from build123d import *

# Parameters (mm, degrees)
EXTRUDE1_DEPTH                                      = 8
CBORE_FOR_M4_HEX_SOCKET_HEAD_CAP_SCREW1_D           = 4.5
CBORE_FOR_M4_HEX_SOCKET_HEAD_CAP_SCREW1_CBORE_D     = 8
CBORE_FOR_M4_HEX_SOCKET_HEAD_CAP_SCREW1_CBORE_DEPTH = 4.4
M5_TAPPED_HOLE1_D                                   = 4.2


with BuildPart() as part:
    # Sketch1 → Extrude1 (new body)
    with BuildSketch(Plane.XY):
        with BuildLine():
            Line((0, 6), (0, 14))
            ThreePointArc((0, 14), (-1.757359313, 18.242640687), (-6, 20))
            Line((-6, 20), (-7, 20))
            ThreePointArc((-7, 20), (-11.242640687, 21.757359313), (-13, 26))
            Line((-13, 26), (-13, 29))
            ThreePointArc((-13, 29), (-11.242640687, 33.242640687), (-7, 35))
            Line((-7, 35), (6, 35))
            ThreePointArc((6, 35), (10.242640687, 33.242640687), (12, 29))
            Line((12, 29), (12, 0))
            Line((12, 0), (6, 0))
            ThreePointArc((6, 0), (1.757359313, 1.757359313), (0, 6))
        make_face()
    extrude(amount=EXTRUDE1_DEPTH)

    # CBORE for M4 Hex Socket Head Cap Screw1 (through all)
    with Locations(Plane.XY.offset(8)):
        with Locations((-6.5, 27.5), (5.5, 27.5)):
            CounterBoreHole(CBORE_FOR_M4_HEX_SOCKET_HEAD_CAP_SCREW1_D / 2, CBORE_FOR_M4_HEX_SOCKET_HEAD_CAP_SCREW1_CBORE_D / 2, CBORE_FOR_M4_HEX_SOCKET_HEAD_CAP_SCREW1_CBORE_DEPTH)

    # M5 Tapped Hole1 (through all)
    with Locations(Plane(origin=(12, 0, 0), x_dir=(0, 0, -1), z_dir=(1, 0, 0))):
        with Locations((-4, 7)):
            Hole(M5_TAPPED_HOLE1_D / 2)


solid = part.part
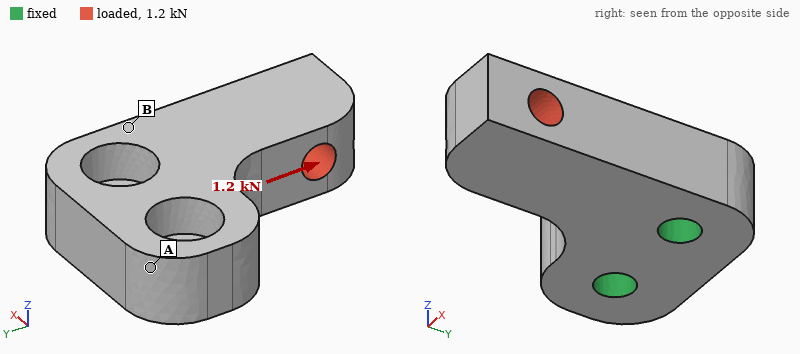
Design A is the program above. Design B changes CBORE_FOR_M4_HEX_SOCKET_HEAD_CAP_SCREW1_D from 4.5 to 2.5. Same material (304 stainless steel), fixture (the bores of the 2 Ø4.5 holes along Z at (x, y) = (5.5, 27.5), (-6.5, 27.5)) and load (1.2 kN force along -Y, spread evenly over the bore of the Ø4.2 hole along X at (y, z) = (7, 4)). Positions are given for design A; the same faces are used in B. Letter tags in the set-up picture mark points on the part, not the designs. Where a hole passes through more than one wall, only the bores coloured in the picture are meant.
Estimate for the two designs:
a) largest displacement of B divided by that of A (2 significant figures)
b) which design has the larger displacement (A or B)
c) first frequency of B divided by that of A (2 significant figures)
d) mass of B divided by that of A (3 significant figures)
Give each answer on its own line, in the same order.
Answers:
1.6
B
0.81
1.02
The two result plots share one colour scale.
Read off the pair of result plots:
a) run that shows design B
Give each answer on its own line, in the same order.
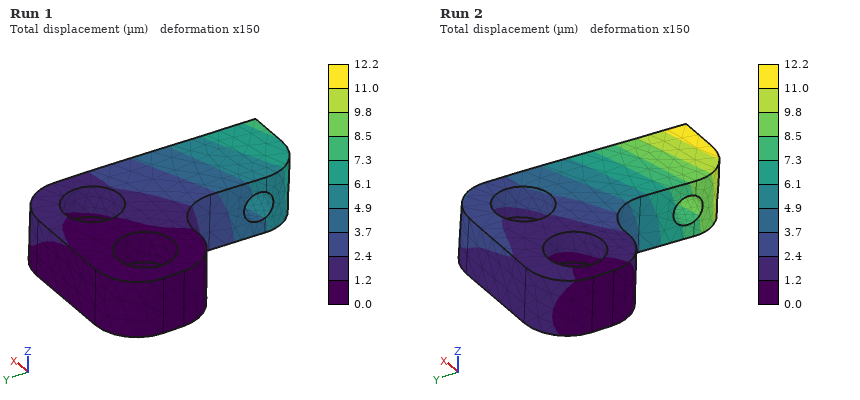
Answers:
Run 2
